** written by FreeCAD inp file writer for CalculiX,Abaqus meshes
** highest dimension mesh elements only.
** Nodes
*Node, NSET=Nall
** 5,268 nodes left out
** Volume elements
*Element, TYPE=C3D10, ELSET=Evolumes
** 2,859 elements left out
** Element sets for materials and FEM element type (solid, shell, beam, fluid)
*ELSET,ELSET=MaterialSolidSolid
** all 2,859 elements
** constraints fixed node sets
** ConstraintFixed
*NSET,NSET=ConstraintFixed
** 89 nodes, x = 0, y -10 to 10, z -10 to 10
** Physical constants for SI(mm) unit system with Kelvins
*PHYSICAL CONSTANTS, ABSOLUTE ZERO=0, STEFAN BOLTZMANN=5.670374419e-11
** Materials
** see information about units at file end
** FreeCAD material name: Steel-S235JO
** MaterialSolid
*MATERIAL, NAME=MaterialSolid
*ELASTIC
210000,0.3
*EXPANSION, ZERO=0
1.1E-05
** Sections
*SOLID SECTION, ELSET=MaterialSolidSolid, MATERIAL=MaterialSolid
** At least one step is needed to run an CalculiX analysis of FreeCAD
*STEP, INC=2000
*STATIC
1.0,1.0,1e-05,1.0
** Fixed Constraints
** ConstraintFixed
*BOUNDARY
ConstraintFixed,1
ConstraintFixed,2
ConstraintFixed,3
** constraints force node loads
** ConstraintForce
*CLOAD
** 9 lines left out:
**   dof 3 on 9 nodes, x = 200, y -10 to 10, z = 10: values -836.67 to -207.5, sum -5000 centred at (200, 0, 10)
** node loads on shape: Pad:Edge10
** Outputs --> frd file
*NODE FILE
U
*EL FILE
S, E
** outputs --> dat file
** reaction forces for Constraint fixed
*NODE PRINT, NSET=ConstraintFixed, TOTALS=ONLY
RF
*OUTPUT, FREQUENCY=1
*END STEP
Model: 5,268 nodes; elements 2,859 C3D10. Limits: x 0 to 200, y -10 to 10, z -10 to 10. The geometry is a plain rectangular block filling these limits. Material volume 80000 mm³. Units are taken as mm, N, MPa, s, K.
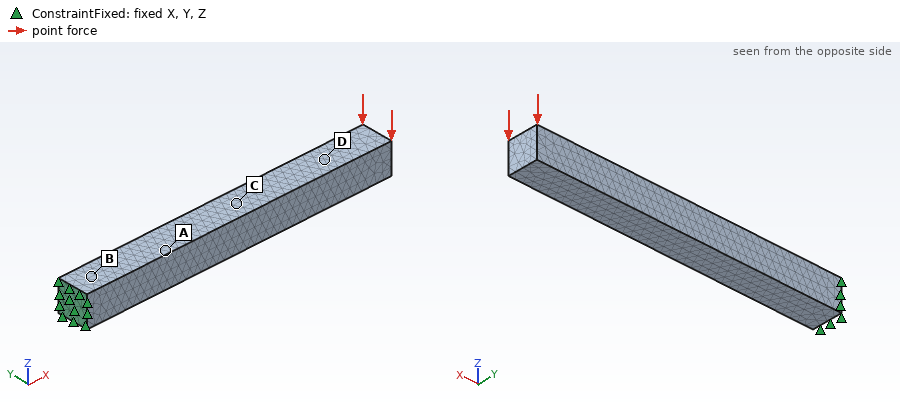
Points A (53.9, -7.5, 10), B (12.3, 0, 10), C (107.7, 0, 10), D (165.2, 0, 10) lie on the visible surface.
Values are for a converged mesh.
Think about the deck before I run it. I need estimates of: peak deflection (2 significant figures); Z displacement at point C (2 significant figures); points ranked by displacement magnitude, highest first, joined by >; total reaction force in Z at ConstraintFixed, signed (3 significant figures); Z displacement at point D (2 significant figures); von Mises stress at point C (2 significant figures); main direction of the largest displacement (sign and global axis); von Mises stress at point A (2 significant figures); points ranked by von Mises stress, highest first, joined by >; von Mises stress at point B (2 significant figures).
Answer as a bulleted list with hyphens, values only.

- 4.8 mm
- -1.7 mm
- D > C > A > B
- 5000 N
- -3.5 mm
- 350 MPa
- -Z
- 550 MPa
- B > A > C > D
- 710 MPa
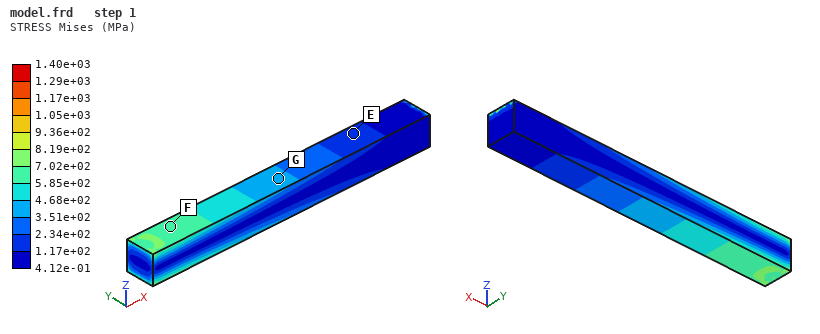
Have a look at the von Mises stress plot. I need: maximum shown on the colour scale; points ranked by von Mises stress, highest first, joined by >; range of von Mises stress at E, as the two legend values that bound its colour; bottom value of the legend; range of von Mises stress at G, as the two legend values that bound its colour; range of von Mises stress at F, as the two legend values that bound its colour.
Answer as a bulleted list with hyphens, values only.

- 1.40e+03 MPa
- F > G > E
- 1.17e+02 to 2.34e+02 MPa
- 4.12e-01 MPa
- 3.51e+02 to 4.68e+02 MPa
- 5.85e+02 to 7.02e+02 MPa
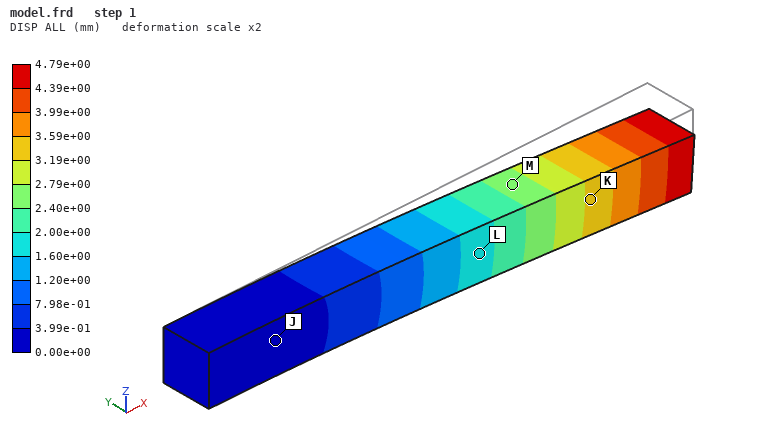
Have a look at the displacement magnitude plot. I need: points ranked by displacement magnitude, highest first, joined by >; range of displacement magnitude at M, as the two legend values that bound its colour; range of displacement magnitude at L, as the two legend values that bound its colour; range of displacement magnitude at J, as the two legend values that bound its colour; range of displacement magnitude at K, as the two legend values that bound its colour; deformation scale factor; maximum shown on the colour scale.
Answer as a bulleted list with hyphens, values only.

- K > M > L > J
- 2.40e+00 to 2.79e+00 mm
- 1.60e+00 to 2.00e+00 mm
- 0.00e+00 to 3.99e-01 mm
- 3.19e+00 to 3.59e+00 mm
- 2
- 4.79e+00 mm
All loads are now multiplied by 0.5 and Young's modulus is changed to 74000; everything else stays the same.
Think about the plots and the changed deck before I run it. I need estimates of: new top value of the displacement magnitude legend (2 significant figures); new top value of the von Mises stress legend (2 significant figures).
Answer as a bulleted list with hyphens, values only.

- 6.8 mm
- 700 MPa
